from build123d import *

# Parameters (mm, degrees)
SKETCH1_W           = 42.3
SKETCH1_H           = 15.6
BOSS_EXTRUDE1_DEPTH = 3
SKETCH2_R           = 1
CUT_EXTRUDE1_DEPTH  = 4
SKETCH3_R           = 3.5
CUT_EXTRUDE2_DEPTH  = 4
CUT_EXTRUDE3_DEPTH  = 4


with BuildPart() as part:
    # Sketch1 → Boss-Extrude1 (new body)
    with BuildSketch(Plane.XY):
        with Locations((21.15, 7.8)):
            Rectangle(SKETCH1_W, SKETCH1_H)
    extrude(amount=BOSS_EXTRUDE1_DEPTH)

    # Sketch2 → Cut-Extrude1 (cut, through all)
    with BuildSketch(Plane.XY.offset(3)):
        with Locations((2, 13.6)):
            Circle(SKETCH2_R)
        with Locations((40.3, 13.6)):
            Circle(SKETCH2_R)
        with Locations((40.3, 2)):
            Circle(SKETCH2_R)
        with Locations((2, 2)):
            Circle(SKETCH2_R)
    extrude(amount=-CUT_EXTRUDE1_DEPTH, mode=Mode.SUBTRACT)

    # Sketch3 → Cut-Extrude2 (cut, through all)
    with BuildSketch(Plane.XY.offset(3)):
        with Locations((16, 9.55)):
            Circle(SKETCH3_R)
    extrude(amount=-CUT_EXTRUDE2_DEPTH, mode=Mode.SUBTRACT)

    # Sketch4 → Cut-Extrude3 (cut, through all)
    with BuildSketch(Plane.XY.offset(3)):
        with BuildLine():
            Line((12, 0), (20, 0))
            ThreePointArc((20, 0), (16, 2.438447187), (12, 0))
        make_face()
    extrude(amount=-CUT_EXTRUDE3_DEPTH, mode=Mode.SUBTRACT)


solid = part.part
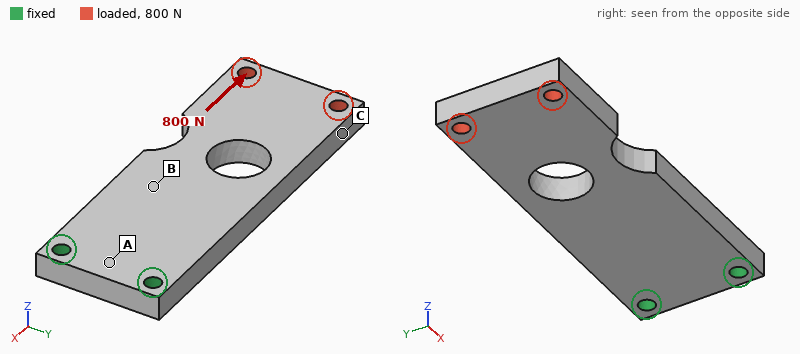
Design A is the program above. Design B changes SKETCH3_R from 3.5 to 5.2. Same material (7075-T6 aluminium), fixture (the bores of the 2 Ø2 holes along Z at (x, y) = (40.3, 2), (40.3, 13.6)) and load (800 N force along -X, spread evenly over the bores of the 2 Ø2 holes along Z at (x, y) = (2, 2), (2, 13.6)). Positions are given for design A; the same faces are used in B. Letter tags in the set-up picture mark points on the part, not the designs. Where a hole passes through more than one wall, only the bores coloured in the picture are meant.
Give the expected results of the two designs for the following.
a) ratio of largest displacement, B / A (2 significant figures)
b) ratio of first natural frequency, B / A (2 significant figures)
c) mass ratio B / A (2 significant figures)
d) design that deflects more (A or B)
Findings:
2.0
0.97
0.92
B
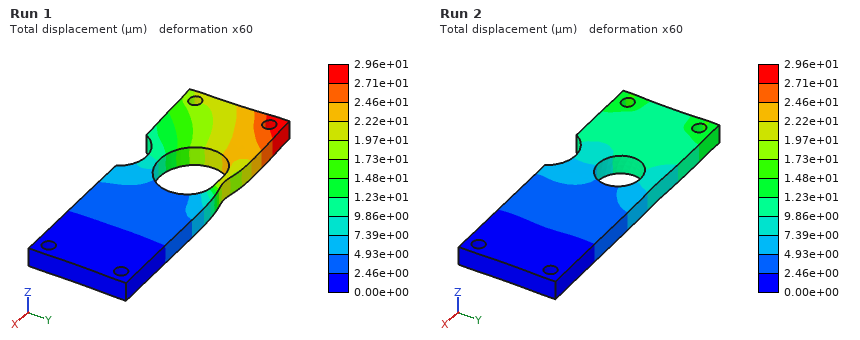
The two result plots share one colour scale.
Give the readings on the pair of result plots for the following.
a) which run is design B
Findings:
Run 1
